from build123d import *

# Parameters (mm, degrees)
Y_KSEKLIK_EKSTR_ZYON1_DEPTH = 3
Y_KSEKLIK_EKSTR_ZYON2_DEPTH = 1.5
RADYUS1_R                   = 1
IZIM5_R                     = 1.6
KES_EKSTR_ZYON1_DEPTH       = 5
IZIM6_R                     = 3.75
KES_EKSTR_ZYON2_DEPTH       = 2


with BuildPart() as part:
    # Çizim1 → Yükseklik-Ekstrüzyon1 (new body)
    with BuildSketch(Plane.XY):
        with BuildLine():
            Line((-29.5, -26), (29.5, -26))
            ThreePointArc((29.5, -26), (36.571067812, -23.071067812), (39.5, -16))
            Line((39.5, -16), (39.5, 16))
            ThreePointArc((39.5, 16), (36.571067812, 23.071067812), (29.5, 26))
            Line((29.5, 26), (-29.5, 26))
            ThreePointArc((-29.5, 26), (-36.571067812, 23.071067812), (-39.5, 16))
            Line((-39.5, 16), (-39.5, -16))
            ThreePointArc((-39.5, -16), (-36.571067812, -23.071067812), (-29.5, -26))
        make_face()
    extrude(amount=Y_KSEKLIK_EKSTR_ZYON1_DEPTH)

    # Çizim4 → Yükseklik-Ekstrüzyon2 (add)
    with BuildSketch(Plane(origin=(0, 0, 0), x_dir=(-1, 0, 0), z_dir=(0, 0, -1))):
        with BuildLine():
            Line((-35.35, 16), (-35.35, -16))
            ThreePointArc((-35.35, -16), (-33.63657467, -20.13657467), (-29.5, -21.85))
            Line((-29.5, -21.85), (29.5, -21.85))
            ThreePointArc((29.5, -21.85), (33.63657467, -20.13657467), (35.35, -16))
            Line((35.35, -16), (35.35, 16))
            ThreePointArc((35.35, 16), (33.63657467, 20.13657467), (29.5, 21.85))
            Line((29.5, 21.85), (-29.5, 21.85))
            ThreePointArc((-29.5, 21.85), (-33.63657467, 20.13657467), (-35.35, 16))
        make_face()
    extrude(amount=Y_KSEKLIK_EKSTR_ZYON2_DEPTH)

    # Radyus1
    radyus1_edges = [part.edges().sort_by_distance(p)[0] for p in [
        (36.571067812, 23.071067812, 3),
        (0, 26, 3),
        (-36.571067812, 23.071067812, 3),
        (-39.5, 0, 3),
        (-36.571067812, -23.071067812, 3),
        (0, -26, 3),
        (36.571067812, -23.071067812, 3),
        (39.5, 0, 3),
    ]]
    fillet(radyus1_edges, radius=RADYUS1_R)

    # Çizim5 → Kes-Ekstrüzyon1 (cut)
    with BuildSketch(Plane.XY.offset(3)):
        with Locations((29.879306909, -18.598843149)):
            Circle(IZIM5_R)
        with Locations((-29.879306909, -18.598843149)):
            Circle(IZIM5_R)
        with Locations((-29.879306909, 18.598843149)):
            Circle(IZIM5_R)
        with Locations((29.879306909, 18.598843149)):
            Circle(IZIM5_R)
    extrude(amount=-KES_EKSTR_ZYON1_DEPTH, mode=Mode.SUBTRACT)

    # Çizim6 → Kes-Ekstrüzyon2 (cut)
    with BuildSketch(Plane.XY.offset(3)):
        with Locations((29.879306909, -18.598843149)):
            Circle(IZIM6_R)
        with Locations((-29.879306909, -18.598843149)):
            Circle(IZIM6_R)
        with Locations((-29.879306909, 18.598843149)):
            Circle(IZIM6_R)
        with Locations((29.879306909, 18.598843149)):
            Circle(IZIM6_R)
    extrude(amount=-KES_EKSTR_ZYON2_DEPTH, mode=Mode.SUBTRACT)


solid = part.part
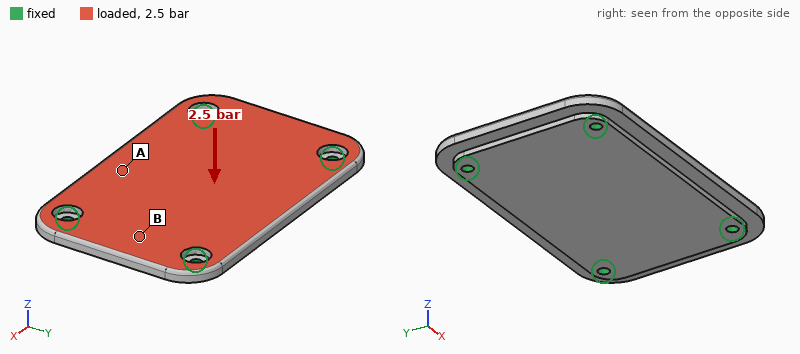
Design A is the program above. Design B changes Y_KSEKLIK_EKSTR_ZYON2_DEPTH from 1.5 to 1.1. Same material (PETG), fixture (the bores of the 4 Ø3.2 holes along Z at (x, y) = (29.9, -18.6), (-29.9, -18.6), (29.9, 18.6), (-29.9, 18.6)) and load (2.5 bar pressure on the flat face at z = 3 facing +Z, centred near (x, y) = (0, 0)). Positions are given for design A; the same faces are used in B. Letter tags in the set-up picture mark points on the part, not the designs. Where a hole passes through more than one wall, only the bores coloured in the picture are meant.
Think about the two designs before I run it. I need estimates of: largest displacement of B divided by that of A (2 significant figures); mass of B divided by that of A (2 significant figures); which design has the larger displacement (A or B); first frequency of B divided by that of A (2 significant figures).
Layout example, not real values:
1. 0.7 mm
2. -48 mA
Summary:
1. 1.3
2. 0.93
3. B
4. 0.91
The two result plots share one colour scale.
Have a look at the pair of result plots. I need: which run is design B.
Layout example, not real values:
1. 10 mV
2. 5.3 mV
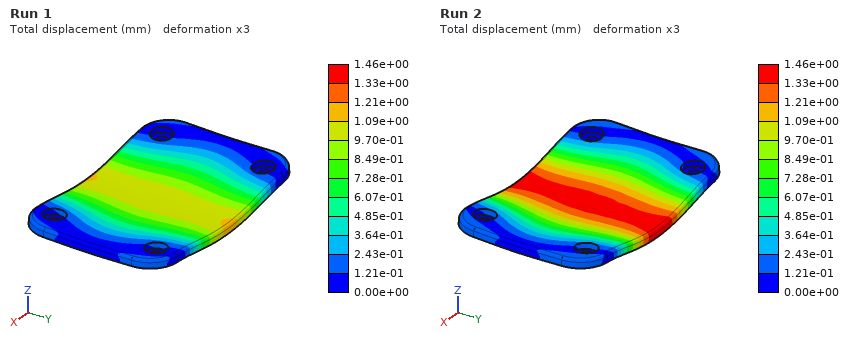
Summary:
1. Run 2
